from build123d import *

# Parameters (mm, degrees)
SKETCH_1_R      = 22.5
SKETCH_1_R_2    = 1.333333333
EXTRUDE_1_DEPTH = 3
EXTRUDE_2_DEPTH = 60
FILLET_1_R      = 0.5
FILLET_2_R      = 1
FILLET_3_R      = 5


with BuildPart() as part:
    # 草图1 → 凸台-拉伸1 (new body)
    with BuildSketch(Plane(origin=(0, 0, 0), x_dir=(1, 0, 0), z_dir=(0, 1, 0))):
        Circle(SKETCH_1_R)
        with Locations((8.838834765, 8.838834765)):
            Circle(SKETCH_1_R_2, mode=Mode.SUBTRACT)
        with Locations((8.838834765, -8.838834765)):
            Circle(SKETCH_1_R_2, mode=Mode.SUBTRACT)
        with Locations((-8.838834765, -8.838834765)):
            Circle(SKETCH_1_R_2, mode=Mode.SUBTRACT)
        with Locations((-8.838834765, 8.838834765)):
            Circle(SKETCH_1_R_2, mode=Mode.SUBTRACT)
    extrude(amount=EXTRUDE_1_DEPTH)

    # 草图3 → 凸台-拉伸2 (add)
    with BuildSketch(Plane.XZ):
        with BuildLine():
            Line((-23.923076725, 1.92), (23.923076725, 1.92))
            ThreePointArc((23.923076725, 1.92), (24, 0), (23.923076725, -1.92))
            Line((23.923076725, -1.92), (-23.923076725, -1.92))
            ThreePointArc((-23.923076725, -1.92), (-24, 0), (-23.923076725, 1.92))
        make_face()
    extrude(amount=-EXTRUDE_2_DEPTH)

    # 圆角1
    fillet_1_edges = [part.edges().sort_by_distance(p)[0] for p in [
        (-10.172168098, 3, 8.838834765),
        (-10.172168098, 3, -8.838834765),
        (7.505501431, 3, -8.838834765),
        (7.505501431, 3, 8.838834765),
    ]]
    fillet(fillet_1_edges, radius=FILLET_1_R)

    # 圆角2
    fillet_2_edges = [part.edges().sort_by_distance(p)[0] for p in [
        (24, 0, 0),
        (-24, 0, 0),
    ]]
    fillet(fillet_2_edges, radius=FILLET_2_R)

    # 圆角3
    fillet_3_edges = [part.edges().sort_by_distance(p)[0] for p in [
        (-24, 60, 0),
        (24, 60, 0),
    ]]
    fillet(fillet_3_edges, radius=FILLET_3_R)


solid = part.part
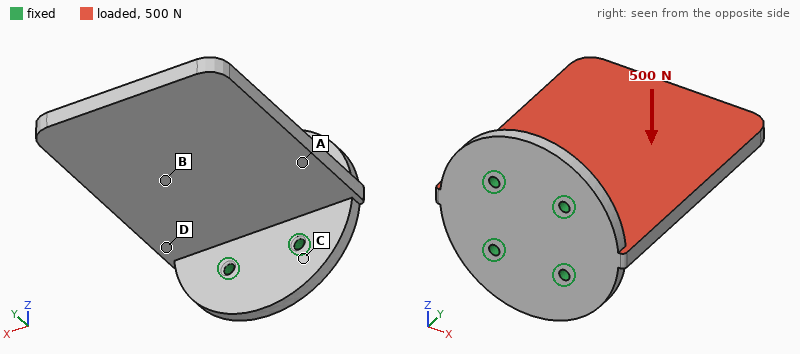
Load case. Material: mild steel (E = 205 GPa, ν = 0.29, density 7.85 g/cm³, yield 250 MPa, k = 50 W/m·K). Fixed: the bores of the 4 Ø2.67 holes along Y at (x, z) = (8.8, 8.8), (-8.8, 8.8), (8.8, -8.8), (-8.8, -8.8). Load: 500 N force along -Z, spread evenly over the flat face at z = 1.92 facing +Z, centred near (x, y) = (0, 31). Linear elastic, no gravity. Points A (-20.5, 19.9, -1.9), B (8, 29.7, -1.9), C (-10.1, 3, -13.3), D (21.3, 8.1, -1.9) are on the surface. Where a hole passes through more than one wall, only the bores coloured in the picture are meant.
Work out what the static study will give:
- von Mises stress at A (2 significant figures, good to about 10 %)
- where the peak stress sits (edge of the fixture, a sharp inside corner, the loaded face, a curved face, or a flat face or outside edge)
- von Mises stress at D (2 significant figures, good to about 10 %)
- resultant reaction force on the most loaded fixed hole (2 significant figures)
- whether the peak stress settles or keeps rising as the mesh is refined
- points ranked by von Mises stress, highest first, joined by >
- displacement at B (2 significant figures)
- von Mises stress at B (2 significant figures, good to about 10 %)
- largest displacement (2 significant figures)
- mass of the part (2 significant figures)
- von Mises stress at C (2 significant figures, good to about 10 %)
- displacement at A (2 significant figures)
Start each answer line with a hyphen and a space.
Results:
- 59 MPa
- edge of the fixture
- 84 MPa
- 530 N
- keeps rising
- D > A > B > C
- 0.11 mm
- 31 MPa
- 0.30 mm
- 120 g
- 19 MPa
- 0.054 mm
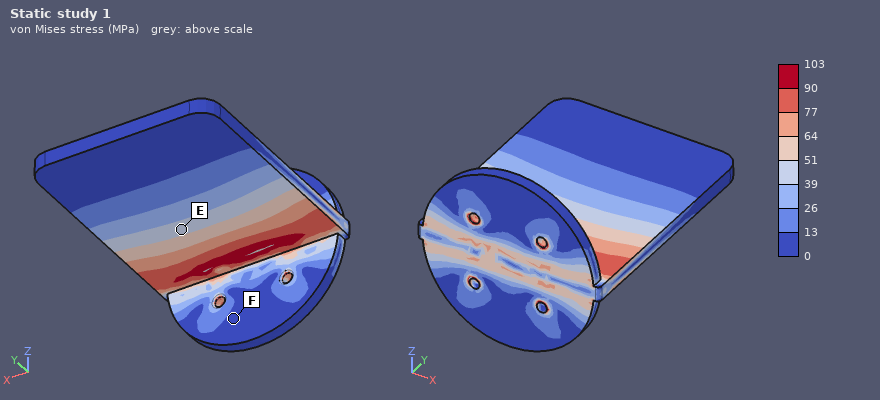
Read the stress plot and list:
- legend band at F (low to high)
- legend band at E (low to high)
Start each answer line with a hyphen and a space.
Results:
- 0 to 13 MPa
- 39 to 51 MPa
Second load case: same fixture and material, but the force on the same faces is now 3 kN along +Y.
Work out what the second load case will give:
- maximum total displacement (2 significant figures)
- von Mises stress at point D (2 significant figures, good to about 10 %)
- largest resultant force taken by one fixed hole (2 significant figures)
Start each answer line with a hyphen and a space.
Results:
- 0.15 mm
- 38 MPa
- 970 N
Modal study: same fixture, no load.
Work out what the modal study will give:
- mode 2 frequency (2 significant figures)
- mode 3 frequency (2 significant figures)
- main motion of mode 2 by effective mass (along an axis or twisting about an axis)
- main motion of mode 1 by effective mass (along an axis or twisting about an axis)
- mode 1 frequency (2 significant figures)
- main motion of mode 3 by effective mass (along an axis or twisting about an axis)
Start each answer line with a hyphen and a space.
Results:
- 2500 Hz
- 2800 Hz
- twisting about Y
- along Z
- 890 Hz
- along X
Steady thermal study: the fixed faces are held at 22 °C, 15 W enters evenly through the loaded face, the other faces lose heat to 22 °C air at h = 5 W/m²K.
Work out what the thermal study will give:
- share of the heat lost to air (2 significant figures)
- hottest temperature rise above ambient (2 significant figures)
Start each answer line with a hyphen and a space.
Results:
- 5.5 %
- 57 K
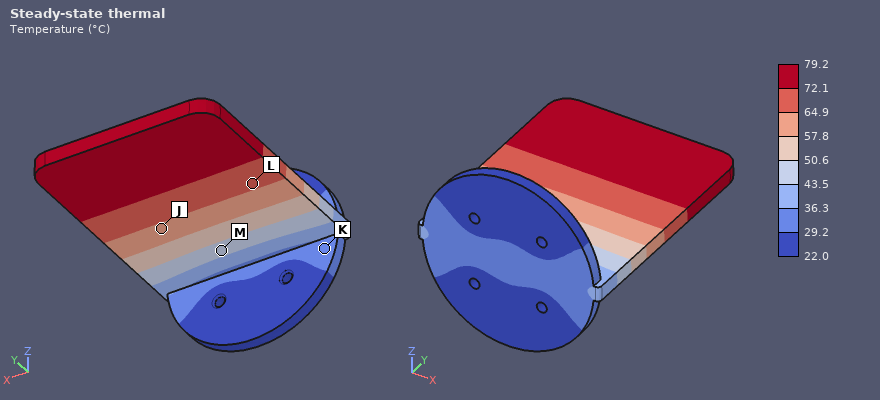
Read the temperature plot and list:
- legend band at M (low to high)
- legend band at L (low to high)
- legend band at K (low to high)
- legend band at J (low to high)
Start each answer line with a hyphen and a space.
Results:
- 43.5 to 50.6 °C
- 64.9 to 72.1 °C
- 29.2 to 36.3 °C
- 57.8 to 64.9 °C
